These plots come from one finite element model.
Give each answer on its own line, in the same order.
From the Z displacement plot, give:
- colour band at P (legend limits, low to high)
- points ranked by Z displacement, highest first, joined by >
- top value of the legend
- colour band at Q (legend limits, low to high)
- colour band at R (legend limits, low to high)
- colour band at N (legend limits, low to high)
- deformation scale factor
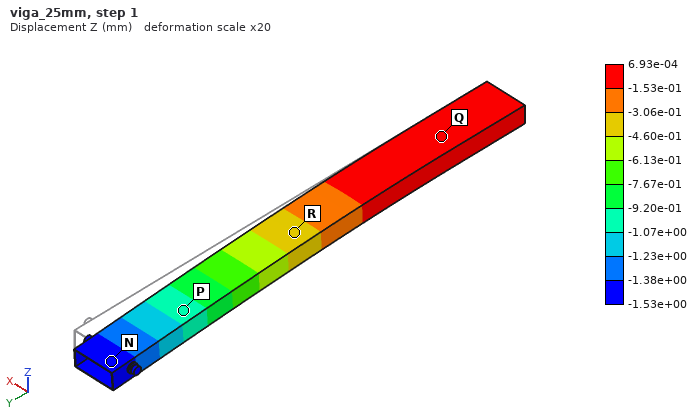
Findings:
-1.07e+00 to -9.20e-01 mm
Q > R > P > N
6.93e-04 mm
-1.53e-01 to 6.93e-04 mm
-4.60e-01 to -3.06e-01 mm
-1.53e+00 to -1.38e+00 mm
20
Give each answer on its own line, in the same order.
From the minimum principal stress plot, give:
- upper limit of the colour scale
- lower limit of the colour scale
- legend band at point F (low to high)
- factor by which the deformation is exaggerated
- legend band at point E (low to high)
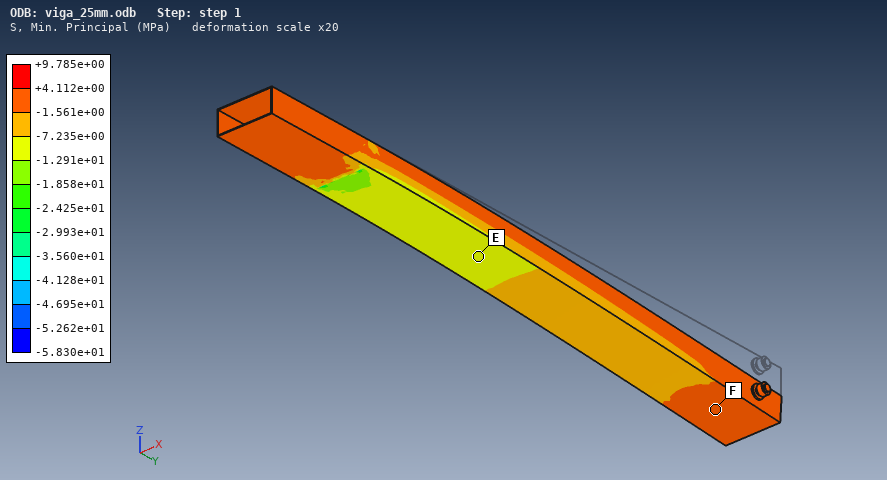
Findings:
+9.785e+00 MPa
-5.830e+01 MPa
-1.561e+00 to +4.112e+00 MPa
20
-1.291e+01 to -7.235e+00 MPa
